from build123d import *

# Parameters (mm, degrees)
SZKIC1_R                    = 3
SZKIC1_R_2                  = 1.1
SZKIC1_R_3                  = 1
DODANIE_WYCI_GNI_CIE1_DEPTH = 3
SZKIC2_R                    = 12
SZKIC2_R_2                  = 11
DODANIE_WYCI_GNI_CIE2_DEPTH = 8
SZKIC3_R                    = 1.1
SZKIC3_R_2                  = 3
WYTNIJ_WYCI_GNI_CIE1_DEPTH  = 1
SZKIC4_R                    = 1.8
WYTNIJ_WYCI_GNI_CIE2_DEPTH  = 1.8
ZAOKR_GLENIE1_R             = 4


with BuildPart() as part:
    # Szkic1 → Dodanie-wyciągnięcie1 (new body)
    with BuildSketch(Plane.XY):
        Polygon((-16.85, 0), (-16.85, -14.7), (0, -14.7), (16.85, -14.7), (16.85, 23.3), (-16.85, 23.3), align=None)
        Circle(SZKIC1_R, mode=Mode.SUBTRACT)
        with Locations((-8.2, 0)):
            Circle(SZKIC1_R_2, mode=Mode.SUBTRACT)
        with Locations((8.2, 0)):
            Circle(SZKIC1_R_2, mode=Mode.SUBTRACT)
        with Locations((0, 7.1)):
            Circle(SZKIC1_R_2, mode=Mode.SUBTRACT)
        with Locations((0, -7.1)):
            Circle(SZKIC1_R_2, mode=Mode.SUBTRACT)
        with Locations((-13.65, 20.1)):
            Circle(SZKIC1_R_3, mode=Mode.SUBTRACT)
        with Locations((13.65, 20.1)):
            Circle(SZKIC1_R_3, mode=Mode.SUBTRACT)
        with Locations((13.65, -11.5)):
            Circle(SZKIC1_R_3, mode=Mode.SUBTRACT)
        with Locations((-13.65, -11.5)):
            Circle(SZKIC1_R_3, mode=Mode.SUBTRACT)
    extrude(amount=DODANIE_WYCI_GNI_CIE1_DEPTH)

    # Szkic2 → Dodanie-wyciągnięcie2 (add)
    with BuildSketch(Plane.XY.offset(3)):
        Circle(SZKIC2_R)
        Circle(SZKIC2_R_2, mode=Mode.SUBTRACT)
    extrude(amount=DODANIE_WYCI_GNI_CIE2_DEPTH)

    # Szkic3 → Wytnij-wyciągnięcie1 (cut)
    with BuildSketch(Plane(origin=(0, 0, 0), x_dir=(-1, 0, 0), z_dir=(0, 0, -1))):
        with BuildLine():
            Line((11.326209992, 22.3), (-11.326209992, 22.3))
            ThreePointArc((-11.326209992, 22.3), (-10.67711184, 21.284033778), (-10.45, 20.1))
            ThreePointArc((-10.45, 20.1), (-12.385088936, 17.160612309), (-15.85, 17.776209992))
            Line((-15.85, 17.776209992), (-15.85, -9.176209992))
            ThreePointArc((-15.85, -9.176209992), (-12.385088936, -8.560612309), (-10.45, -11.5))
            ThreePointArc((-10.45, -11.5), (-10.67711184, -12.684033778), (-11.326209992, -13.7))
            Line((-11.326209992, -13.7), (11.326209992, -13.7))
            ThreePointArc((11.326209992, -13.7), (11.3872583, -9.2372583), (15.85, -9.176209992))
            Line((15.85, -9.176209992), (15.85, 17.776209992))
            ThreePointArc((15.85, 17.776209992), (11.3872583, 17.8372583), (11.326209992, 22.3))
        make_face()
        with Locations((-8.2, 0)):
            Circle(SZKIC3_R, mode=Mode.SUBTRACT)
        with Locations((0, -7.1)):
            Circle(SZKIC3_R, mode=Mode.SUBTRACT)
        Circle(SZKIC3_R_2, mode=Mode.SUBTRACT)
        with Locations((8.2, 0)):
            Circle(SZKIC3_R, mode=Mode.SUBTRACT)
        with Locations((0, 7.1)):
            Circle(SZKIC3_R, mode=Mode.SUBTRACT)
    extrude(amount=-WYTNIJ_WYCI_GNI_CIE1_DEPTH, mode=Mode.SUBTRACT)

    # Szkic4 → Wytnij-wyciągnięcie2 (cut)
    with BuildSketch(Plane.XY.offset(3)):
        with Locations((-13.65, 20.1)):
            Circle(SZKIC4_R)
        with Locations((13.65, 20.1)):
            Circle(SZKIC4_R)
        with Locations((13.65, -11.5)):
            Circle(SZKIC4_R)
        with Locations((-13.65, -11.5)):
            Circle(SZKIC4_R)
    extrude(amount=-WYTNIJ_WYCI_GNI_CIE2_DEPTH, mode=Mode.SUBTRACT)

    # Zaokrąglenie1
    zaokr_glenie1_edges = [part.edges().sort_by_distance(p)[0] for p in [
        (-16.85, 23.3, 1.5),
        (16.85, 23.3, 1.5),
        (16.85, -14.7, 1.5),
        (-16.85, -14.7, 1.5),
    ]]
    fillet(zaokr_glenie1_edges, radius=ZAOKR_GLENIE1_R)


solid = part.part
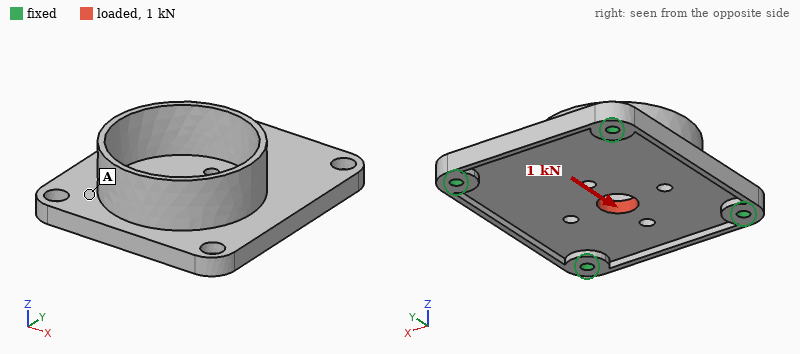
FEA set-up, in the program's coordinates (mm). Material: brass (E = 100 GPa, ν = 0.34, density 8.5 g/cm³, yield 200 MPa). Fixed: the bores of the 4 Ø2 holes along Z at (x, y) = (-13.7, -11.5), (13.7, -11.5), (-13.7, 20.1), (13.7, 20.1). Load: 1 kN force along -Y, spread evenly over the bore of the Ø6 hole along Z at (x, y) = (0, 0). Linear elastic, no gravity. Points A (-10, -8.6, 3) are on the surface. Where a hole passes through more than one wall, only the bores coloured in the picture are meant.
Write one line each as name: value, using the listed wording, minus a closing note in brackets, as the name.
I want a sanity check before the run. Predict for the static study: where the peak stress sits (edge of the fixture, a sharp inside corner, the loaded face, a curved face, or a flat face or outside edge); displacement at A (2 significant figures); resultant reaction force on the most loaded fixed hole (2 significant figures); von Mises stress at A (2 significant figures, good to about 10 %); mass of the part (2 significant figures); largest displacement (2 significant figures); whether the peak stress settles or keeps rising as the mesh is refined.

where the peak stress sits: edge of the fixture
displacement at A: 3.4 µm
resultant reaction force on the most loaded fixed hole: 270 N
von Mises stress at A: 8.9 MPa
mass of the part: 27 g
largest displacement: 6.2 µm
whether the peak stress settles or keeps rising as the mesh is refined: keeps rising
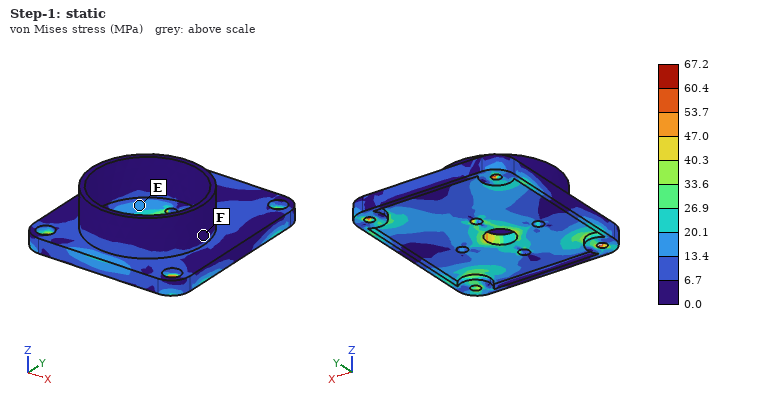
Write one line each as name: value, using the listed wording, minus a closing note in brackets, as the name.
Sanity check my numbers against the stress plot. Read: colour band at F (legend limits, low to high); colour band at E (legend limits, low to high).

colour band at F: 0.0 to 6.7 MPa
colour band at E: 13.4 to 20.1 MPa
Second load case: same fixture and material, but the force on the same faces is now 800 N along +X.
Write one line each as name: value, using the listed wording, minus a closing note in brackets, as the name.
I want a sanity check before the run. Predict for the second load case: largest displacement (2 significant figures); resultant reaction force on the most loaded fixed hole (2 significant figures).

largest displacement: 5.0 µm
resultant reaction force on the most loaded fixed hole: 250 N
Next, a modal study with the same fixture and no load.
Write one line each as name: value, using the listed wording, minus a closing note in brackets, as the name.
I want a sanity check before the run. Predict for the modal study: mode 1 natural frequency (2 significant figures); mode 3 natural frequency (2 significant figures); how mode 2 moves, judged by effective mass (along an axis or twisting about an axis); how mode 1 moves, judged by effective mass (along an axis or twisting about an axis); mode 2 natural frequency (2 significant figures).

mode 1 natural frequency: 5700 Hz
mode 3 natural frequency: 8900 Hz
how mode 2 moves, judged by effective mass: twisting about Y
how mode 1 moves, judged by effective mass: along Z
mode 2 natural frequency: 7900 Hz
